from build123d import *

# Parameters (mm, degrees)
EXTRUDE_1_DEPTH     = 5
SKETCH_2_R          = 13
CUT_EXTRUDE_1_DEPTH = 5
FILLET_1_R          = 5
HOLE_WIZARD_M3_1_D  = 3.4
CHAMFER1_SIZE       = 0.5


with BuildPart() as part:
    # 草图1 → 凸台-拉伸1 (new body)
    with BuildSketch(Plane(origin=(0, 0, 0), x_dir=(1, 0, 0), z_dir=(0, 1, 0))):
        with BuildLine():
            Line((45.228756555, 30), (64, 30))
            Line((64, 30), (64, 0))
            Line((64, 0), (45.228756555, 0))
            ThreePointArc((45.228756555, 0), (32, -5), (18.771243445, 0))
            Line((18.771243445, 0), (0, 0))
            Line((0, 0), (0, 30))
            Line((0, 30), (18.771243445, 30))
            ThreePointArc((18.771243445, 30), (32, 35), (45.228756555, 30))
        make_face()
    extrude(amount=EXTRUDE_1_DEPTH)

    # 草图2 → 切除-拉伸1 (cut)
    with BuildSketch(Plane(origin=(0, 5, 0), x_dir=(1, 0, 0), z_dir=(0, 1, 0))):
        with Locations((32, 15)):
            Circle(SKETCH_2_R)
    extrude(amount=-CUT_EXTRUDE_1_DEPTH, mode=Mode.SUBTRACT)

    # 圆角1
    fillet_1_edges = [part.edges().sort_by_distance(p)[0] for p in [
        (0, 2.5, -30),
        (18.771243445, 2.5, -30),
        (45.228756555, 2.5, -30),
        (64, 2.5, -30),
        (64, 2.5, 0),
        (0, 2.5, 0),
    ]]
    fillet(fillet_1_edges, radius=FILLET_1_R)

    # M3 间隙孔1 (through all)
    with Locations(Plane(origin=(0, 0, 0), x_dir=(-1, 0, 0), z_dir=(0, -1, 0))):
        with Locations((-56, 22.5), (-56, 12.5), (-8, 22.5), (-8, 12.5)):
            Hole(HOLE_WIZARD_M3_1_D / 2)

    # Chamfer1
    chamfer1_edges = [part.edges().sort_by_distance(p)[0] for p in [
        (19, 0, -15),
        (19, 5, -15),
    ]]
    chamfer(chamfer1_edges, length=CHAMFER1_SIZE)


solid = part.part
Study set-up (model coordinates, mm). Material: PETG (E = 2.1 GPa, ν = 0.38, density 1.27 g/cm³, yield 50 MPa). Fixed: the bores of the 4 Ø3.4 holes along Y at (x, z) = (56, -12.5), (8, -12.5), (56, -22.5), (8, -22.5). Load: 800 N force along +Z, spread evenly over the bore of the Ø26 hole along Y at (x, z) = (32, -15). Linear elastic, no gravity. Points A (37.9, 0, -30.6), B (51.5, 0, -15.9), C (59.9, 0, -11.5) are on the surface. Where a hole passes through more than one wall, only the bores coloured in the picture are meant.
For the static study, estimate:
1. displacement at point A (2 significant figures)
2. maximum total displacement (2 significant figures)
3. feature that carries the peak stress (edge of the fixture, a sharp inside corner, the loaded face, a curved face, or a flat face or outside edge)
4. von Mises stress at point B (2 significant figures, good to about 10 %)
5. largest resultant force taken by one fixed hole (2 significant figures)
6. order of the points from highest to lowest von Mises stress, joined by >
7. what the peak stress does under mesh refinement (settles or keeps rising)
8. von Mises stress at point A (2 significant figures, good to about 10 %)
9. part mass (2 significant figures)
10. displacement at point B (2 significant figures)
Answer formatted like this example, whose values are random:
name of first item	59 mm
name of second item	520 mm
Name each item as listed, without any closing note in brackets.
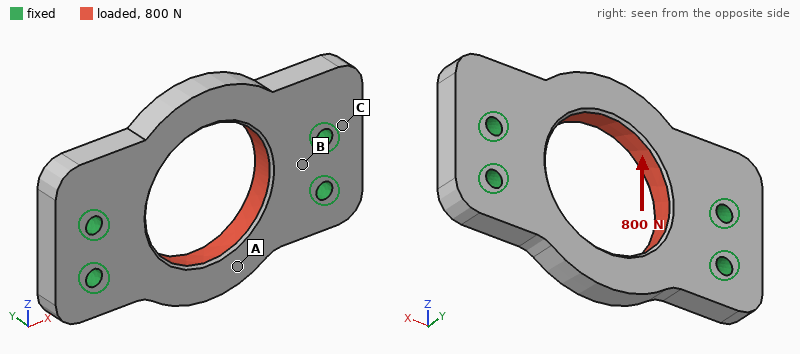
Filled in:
displacement at point A	0.096 mm
maximum total displacement	0.11 mm
feature that carries the peak stress	edge of the fixture
von Mises stress at point B	8.3 MPa
largest resultant force taken by one fixed hole	250 N
order of the points from highest to lowest von Mises stress, joined by >	B > A > C
what the peak stress does under mesh refinement	keeps rising
von Mises stress at point A	4.9 MPa
part mass	9.6 g
displacement at point B	0.021 mm
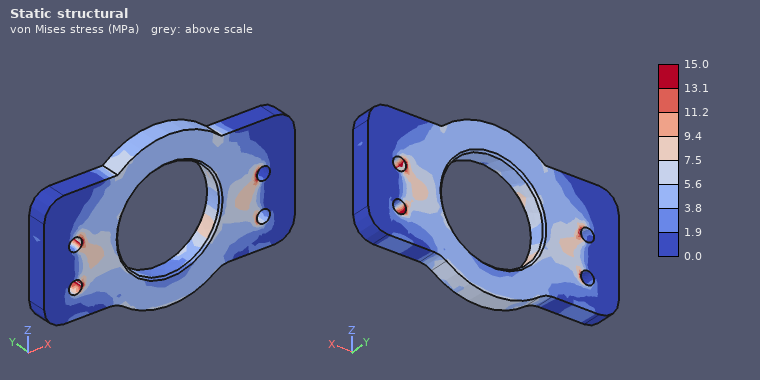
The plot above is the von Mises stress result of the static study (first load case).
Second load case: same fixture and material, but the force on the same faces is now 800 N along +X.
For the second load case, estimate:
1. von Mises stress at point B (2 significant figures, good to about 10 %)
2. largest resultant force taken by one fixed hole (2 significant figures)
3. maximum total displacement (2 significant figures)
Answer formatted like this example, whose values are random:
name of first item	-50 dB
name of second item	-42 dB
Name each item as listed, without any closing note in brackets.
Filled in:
von Mises stress at point B	2.2 MPa
largest resultant force taken by one fixed hole	250 N
maximum total displacement	68 µm
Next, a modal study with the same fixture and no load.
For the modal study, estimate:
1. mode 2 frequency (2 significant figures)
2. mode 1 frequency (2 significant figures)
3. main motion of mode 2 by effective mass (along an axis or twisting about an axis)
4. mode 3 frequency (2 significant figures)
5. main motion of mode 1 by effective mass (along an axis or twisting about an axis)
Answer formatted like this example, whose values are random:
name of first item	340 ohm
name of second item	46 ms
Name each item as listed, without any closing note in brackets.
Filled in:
mode 2 frequency	2700 Hz
mode 1 frequency	2200 Hz
main motion of mode 2 by effective mass	along Y
mode 3 frequency	5100 Hz
main motion of mode 1 by effective mass	along Y
